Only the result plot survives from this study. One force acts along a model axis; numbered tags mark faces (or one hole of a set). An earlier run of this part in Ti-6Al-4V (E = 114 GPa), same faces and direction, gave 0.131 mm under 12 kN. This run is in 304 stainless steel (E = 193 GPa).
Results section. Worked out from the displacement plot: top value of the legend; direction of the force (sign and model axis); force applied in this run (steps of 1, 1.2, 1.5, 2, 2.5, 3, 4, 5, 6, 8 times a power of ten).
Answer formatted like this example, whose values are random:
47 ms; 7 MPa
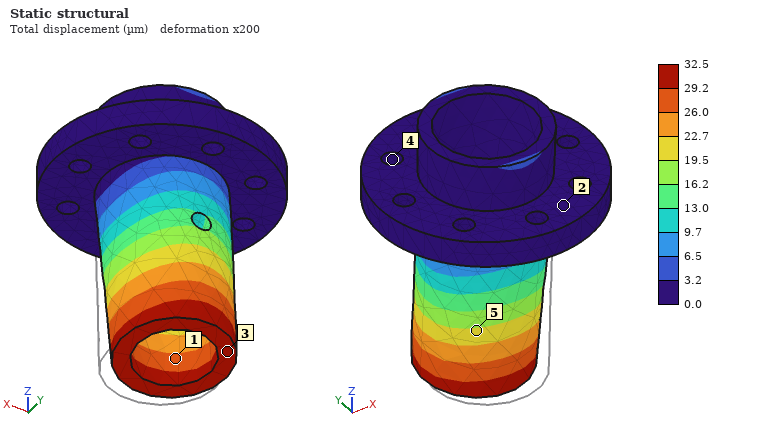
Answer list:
32.5 µm; +Y; 5 kN
